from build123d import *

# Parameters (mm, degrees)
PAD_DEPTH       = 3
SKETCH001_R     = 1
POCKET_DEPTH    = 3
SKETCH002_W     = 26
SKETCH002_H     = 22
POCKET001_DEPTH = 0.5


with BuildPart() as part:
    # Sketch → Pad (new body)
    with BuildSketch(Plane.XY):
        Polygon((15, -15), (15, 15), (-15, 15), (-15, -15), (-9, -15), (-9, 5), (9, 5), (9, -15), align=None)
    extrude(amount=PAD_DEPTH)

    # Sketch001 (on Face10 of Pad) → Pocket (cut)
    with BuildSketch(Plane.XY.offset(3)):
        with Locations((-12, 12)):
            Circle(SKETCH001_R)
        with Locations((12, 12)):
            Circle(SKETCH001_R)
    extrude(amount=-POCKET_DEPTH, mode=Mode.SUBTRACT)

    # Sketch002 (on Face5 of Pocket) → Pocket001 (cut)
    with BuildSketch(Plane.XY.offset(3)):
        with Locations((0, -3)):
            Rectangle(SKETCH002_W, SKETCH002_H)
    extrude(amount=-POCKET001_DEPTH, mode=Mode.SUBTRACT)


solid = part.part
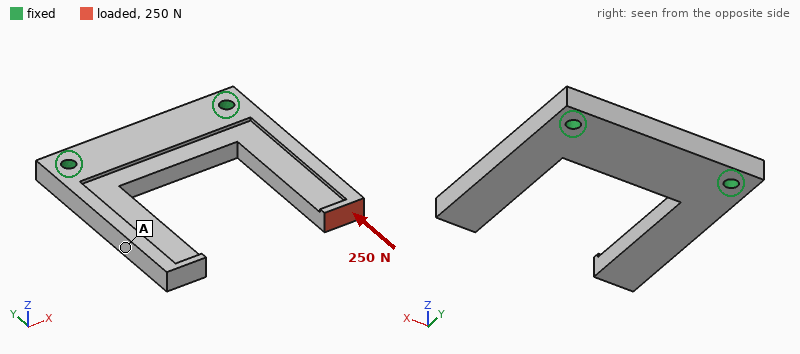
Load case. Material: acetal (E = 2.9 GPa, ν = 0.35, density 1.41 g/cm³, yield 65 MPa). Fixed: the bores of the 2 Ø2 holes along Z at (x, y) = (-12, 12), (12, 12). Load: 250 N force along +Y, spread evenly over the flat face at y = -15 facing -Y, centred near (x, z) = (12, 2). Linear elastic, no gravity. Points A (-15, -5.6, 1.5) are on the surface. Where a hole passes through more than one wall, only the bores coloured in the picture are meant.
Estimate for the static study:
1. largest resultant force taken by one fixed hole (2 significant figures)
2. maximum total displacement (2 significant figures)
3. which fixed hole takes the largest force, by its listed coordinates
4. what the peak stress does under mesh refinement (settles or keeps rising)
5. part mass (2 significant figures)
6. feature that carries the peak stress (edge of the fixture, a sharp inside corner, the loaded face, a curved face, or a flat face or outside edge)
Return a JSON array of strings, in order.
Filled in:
["250 N", "0.44 mm", "(12, 12)", "keeps rising", "2.1 g", "edge of the fixture"]
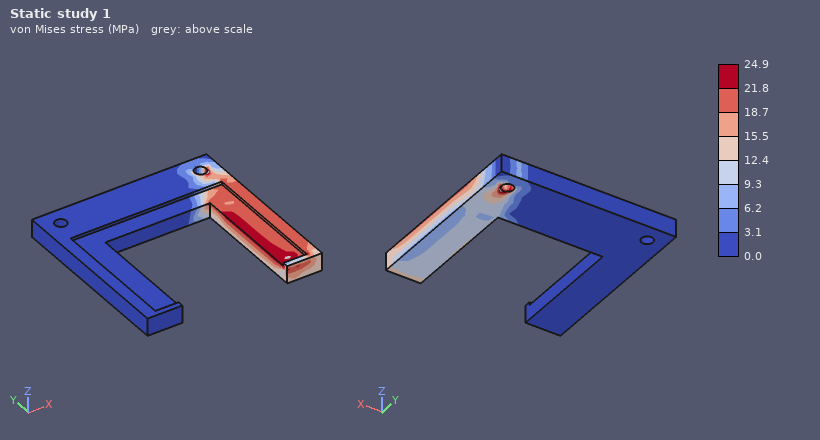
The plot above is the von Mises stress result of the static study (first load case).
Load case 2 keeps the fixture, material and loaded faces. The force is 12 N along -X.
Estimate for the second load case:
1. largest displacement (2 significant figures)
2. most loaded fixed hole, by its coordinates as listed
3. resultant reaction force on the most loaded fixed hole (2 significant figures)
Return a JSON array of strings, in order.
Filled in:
["0.42 mm", "(-12, 12)", "22 N"]
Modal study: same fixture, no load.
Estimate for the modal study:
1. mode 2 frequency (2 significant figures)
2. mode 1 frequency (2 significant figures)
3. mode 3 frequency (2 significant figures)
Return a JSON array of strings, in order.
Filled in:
["1000 Hz", "980 Hz", "2300 Hz"]
